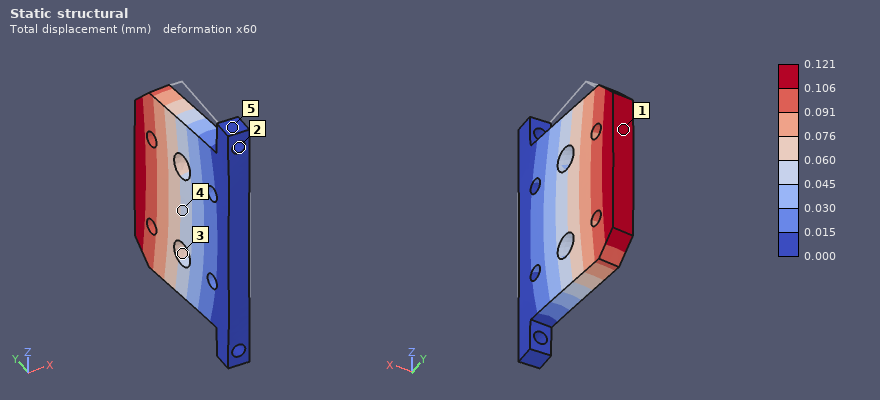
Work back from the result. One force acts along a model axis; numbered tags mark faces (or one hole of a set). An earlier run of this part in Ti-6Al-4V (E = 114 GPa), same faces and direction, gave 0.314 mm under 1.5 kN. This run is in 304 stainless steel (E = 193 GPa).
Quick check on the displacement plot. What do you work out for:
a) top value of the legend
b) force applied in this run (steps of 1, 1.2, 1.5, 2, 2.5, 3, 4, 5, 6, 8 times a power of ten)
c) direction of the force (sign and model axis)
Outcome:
0.121 mm
1 kN
-X
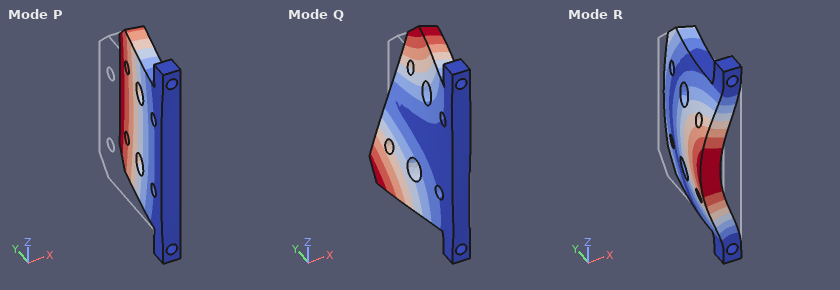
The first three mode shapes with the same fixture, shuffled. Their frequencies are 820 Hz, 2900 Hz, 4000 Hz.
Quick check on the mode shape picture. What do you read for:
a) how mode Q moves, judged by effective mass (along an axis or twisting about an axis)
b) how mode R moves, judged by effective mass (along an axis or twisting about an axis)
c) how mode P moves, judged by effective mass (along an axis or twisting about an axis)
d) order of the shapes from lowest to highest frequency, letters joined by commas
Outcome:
twisting about Y
along X
along X
P, Q, R
